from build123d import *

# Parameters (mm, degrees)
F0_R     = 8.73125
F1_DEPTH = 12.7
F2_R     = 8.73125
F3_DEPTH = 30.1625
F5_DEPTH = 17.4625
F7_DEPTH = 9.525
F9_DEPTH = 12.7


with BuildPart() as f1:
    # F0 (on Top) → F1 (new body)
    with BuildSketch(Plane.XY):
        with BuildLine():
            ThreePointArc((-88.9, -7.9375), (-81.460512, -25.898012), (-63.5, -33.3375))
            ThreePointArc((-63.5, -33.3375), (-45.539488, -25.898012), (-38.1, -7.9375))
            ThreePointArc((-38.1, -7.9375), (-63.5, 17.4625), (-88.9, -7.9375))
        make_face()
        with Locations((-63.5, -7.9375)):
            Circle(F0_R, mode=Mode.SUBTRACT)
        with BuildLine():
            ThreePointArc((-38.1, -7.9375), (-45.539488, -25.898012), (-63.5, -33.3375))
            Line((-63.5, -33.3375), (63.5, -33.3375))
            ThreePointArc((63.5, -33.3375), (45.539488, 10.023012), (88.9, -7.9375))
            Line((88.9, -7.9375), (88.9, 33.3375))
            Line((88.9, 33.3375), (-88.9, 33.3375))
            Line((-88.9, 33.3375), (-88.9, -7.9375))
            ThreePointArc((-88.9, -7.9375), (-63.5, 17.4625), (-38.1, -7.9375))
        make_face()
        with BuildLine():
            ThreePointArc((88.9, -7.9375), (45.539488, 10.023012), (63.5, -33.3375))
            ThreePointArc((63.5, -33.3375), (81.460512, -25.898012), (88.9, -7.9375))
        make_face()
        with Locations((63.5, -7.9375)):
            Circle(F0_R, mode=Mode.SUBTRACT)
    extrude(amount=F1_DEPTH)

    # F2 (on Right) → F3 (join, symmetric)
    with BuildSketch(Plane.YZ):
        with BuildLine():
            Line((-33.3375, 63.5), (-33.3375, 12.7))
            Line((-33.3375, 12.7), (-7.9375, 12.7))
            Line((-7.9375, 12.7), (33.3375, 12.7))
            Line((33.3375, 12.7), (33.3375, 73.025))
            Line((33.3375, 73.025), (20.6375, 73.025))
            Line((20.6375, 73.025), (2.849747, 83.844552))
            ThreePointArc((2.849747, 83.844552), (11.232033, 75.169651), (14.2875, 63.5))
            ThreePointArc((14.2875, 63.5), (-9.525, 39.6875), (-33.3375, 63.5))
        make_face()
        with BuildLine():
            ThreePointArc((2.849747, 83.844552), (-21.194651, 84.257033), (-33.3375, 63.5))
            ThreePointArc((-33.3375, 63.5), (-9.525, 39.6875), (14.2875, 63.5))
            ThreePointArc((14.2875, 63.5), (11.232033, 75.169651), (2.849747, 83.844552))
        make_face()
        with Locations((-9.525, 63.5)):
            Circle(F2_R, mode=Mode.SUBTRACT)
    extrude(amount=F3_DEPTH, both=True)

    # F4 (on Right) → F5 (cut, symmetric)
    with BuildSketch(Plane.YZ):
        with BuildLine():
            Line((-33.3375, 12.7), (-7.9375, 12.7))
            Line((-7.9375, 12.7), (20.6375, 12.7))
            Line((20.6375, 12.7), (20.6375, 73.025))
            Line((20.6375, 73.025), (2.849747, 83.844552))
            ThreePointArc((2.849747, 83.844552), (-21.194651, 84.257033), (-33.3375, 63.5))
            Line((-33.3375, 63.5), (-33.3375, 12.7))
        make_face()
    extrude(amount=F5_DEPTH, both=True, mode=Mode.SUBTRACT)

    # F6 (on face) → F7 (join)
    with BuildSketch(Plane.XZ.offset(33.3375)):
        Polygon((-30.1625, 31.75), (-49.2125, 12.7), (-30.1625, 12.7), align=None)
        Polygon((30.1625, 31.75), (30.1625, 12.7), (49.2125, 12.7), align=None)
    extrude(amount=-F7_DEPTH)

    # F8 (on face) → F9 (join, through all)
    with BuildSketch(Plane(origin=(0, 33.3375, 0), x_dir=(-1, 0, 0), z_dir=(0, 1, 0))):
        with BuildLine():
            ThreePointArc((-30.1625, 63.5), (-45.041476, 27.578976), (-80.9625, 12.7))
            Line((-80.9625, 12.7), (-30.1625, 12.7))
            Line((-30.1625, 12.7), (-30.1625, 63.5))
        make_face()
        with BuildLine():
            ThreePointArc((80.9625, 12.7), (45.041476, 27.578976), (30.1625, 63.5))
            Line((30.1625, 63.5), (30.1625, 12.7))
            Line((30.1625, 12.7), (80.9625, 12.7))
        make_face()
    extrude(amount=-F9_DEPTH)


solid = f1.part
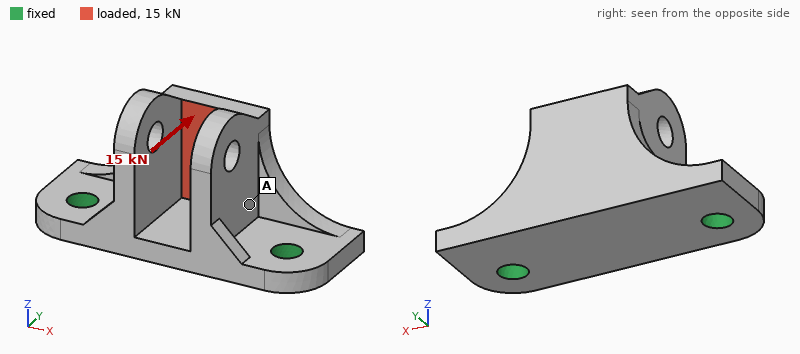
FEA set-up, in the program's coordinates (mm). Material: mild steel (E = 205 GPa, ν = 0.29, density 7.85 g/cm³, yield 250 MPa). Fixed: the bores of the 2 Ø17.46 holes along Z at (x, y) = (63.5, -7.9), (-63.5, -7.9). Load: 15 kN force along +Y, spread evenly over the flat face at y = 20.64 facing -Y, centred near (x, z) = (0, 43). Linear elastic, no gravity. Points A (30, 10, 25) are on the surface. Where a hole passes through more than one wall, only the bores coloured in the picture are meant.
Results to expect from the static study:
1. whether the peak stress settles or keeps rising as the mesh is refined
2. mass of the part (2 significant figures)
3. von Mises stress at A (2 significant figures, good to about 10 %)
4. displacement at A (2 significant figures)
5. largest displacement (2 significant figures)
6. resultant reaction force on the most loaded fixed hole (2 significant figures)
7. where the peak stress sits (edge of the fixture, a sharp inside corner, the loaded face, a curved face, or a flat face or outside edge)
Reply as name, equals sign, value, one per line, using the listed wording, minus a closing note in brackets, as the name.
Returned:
whether the peak stress settles or keeps rising as the mesh is refined = keeps rising
mass of the part = 2.3 kg
von Mises stress at A = 23 MPa
displacement at A = 0.042 mm
largest displacement = 0.13 mm
resultant reaction force on the most loaded fixed hole = 7.8 kN
where the peak stress sits = edge of the fixture
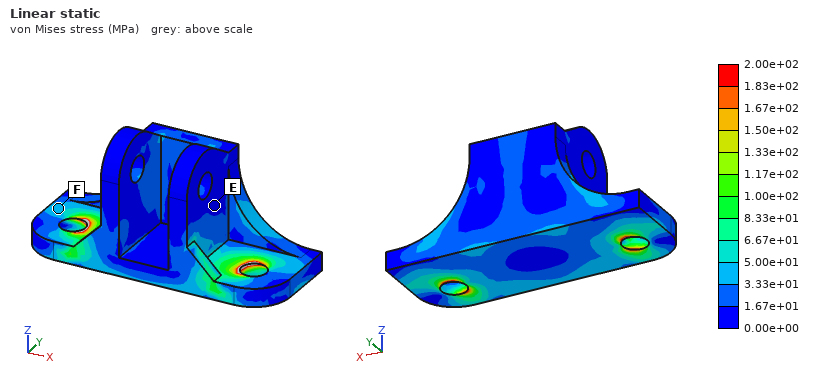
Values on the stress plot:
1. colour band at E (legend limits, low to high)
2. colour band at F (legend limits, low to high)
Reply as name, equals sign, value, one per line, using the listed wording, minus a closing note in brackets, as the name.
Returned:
colour band at E = 0.00e+00 to 1.67e+01 MPa
colour band at F = 3.33e+01 to 5.00e+01 MPa
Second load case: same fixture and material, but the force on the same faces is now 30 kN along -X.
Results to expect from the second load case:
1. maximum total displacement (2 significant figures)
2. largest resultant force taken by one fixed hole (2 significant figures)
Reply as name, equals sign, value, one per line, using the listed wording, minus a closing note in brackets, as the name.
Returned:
maximum total displacement = 77 µm
largest resultant force taken by one fixed hole = 19 kN
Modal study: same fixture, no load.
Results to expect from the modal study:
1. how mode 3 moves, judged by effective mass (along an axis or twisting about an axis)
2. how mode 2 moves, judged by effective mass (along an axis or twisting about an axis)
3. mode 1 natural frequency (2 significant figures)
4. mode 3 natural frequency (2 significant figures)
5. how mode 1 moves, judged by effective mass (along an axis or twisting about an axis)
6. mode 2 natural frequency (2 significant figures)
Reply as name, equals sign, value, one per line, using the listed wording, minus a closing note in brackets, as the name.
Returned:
how mode 3 moves, judged by effective mass = along Z
how mode 2 moves, judged by effective mass = along X
mode 1 natural frequency = 1700 Hz
mode 3 natural frequency = 3200 Hz
how mode 1 moves, judged by effective mass = along Y
mode 2 natural frequency = 3000 Hz
